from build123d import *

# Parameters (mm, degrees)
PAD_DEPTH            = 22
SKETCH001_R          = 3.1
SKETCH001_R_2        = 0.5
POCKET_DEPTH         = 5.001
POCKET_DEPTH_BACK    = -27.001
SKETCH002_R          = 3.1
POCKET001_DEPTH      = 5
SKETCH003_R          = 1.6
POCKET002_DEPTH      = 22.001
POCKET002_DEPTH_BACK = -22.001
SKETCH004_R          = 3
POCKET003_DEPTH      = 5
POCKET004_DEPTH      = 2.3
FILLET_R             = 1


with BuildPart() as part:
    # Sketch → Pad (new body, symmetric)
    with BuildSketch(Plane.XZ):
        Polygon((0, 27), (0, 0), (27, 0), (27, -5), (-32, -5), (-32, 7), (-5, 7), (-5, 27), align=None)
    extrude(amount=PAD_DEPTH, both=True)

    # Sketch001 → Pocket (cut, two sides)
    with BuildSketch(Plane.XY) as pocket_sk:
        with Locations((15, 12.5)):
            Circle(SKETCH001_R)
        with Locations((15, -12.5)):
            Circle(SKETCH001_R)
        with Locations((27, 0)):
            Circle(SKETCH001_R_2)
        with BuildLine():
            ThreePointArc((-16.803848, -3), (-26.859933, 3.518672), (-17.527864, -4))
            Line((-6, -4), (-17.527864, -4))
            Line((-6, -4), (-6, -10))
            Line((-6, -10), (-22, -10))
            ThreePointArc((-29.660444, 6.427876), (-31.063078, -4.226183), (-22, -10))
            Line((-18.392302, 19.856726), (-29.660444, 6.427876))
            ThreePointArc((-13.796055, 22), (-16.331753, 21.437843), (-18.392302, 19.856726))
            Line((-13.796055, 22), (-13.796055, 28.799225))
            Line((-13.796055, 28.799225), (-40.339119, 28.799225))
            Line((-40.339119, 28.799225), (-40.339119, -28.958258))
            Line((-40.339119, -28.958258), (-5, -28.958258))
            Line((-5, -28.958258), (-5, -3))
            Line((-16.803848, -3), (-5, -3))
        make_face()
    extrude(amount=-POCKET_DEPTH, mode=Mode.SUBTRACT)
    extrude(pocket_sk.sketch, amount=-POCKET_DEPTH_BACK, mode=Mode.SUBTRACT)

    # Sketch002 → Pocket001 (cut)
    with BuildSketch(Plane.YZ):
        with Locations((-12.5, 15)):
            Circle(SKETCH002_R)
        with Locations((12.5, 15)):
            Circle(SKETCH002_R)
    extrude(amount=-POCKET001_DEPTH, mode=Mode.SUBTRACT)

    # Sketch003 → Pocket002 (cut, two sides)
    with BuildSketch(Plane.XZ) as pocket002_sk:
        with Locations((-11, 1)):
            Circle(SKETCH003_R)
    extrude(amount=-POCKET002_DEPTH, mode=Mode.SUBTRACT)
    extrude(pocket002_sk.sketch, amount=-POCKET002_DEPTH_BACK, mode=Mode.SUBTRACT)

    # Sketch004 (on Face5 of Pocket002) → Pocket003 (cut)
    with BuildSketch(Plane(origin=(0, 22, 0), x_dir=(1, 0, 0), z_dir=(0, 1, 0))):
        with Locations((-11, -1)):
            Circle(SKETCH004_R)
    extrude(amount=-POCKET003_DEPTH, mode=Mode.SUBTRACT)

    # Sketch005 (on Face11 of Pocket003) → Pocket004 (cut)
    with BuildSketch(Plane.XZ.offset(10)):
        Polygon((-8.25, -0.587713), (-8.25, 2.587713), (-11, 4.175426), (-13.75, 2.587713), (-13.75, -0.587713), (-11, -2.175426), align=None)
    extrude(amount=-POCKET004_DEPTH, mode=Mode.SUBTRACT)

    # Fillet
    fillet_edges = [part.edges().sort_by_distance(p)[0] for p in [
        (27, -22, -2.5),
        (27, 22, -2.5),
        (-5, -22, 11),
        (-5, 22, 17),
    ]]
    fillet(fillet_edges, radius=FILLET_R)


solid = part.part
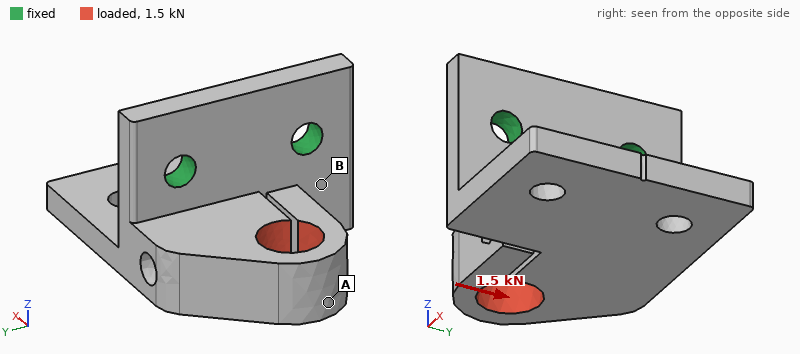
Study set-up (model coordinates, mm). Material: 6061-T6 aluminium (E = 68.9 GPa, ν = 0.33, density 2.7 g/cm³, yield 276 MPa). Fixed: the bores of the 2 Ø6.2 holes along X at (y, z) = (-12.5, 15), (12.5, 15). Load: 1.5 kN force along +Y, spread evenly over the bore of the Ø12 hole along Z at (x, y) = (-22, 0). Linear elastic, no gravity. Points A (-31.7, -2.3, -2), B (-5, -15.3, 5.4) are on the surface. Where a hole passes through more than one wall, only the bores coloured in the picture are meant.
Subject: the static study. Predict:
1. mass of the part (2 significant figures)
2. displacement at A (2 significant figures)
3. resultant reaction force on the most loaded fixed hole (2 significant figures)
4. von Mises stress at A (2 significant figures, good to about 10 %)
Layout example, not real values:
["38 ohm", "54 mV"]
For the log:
["51 g", "0.064 mm", "1.4 kN", "82 MPa"]
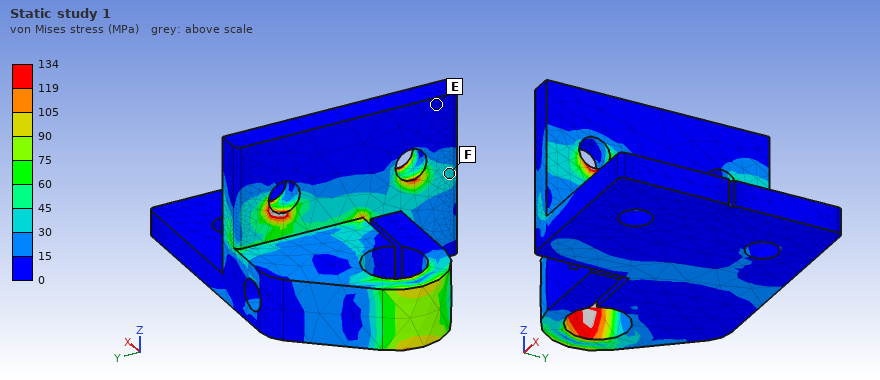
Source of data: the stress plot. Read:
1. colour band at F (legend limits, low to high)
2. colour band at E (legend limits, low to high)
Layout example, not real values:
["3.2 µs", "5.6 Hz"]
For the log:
["30 to 45 MPa", "0 to 15 MPa"]
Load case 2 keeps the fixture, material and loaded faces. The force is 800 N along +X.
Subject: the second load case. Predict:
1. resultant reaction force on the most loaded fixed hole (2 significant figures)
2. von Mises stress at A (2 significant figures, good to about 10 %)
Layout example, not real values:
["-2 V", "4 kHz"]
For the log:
["410 N", "24 MPa"]
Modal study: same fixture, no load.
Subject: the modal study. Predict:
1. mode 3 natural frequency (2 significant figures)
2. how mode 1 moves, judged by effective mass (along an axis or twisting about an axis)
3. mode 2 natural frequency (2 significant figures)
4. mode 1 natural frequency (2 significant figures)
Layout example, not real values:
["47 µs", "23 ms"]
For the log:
["3200 Hz", "along X", "2500 Hz", "2300 Hz"]
